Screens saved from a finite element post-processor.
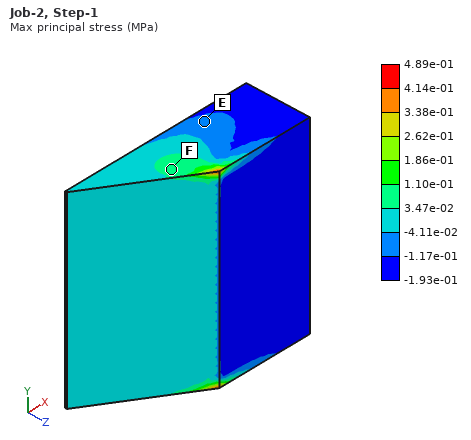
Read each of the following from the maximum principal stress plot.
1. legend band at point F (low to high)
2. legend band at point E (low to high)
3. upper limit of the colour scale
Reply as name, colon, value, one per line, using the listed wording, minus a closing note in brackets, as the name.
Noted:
legend band at point F: 3.47e-02 to 1.10e-01 MPa
legend band at point E: -1.17e-01 to -4.11e-02 MPa
upper limit of the colour scale: 4.89e-01 MPa
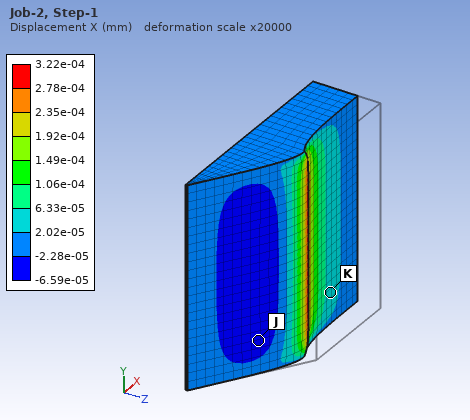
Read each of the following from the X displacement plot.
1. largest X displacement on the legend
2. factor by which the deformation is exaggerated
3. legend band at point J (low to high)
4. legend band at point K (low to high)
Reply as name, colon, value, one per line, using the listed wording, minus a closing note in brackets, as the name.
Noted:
largest X displacement on the legend: 3.22e-04 mm
factor by which the deformation is exaggerated: 20000
legend band at point J: -6.59e-05 to -2.28e-05 mm
legend band at point K: 2.02e-05 to 6.33e-05 mm
